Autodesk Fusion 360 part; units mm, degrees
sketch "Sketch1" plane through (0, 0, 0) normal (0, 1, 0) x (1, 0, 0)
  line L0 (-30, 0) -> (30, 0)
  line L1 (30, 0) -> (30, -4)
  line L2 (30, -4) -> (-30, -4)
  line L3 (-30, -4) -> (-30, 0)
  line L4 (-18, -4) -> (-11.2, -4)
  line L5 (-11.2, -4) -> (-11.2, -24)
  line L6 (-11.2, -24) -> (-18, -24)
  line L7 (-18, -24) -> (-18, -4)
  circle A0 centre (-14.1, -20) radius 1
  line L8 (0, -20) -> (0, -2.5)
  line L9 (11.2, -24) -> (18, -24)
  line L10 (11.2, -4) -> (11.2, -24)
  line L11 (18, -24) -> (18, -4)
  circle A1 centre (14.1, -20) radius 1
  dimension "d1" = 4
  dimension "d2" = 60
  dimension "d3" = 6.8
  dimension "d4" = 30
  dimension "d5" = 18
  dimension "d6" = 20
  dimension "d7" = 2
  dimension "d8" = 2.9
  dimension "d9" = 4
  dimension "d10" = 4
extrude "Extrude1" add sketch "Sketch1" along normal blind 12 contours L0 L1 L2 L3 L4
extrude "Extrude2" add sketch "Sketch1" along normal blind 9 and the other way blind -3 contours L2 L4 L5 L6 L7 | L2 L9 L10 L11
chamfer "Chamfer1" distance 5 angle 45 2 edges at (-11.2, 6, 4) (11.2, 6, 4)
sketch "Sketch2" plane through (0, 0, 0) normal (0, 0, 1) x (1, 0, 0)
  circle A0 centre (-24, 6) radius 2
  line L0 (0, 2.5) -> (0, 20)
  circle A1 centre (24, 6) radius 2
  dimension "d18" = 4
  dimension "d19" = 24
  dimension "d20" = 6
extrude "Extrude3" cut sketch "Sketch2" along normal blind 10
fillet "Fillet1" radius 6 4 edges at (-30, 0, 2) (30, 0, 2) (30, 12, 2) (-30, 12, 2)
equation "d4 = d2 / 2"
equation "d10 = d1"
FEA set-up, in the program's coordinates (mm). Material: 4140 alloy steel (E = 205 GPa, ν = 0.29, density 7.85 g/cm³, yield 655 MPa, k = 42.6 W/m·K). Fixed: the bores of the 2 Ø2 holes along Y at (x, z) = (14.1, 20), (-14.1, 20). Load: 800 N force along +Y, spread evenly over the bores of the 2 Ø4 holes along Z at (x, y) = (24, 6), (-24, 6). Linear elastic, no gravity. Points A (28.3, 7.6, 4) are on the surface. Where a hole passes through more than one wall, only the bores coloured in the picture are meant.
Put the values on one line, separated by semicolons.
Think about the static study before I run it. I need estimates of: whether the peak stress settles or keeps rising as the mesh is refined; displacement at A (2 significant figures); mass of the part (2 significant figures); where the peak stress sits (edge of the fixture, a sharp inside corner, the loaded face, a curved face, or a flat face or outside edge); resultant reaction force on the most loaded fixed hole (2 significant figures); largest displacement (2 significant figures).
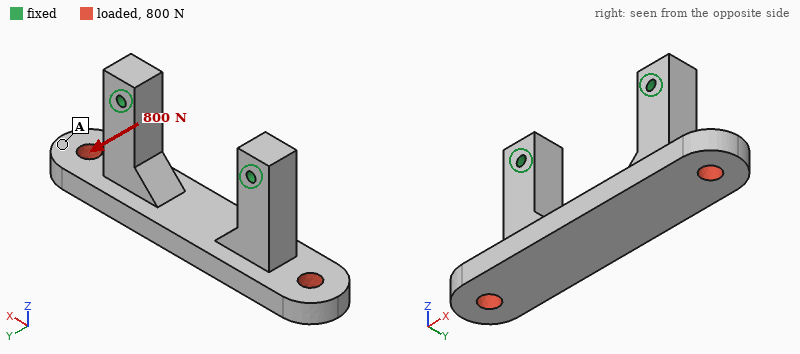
keeps rising; 37 µm; 35 g; edge of the fixture; 400 N; 49 µm
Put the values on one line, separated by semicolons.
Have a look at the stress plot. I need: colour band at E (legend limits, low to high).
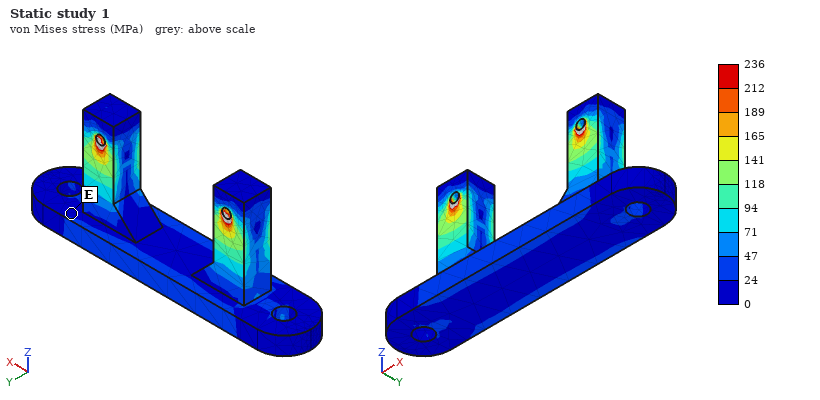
0 to 24 MPa
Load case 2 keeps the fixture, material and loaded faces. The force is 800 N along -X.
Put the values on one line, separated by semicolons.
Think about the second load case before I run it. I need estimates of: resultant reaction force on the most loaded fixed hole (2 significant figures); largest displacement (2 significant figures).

490 N; 18 µm
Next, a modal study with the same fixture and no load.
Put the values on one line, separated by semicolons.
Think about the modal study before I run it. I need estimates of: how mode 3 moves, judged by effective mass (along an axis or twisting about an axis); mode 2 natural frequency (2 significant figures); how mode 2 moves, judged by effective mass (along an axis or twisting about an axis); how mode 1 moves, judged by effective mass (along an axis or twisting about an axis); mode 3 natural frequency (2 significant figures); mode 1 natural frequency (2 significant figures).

along X; 6400 Hz; twisting about Z; along Y; 7600 Hz; 4900 Hz
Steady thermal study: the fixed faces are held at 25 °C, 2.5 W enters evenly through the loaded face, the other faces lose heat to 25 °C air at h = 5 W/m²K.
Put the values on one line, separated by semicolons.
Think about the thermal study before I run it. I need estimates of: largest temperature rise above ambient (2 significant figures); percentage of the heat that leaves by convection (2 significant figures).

18 K; 5.3 %
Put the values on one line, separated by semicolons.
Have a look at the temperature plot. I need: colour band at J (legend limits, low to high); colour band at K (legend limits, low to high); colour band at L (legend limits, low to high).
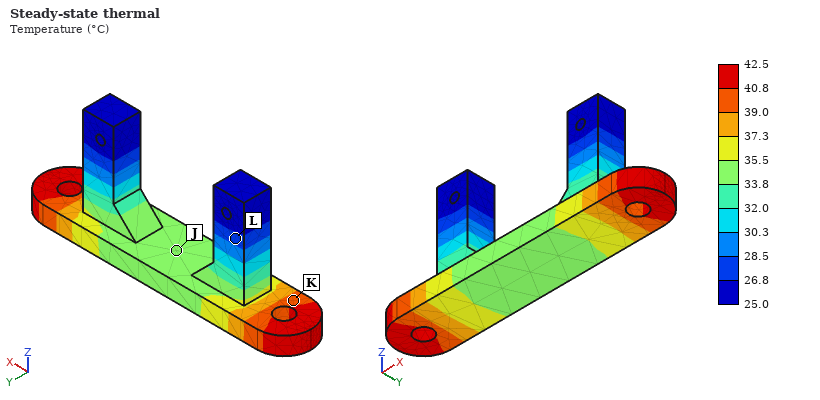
33.8 to 35.5 °C; 39.0 to 40.8 °C; 26.8 to 28.5 °C
